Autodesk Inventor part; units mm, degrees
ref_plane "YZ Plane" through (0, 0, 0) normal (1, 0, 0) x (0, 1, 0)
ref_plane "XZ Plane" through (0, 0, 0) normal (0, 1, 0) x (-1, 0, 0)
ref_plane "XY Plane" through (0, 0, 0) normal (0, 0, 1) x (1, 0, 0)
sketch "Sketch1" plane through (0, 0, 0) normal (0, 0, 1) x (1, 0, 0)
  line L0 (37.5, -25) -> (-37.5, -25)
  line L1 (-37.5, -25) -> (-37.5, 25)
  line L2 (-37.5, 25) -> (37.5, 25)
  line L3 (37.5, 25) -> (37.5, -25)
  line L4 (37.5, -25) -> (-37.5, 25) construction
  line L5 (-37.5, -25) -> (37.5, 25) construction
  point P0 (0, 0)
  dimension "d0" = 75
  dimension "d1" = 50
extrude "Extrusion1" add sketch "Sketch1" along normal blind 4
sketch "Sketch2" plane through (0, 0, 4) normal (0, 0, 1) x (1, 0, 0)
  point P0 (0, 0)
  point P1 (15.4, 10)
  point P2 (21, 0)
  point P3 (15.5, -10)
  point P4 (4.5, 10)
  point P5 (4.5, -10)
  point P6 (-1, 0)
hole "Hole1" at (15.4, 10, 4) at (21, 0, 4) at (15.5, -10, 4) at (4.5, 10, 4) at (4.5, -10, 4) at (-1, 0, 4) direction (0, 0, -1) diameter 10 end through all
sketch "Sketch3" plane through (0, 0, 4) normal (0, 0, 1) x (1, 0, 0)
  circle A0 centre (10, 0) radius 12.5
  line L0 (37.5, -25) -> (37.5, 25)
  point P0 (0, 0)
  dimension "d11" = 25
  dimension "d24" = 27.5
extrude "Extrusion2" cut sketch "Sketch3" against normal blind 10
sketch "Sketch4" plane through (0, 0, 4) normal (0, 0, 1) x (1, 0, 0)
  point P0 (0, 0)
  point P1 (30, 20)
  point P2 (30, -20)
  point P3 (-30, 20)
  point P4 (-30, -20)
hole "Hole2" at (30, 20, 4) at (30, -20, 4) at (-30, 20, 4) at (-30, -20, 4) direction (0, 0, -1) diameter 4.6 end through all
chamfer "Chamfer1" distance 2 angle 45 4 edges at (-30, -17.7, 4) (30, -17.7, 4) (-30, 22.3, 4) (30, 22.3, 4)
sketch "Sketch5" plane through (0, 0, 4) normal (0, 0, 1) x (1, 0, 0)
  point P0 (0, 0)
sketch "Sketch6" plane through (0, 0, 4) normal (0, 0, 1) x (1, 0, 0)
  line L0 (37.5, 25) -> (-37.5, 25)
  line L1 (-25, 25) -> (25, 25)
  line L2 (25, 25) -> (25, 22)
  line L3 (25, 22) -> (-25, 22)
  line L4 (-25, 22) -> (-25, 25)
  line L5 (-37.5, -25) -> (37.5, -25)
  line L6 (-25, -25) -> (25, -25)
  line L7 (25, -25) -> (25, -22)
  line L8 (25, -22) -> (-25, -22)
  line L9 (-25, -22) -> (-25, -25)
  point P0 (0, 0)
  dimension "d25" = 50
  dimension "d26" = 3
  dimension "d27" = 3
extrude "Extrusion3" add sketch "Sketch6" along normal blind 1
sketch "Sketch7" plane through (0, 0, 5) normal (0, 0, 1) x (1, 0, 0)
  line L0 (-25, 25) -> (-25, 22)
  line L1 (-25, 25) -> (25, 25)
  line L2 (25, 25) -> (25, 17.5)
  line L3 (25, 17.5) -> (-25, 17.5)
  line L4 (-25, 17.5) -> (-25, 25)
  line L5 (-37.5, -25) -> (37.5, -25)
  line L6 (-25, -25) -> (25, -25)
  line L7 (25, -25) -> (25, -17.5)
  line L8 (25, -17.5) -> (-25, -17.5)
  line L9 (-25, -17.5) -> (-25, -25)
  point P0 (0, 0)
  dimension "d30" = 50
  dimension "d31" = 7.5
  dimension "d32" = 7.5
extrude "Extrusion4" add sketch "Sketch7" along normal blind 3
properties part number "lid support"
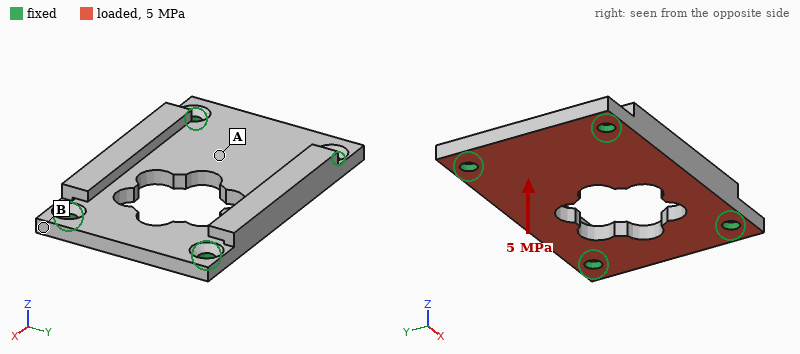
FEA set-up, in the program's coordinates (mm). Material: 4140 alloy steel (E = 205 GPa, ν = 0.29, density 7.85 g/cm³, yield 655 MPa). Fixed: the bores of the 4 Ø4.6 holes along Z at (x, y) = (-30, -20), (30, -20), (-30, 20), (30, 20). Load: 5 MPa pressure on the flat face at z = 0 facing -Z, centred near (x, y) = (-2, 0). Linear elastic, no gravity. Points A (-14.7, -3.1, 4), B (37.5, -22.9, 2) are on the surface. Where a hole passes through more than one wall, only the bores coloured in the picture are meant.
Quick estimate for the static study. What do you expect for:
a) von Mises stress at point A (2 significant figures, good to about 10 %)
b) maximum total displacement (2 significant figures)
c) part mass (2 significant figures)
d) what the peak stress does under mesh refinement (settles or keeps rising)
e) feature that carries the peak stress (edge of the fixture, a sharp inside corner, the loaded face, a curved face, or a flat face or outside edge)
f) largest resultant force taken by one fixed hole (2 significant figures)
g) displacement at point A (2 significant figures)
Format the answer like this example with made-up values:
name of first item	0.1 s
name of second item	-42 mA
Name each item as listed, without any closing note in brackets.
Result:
von Mises stress at point A	190 MPa
maximum total displacement	0.20 mm
part mass	110 g
what the peak stress does under mesh refinement	keeps rising
feature that carries the peak stress	edge of the fixture
largest resultant force taken by one fixed hole	5.1 kN
displacement at point A	0.14 mm
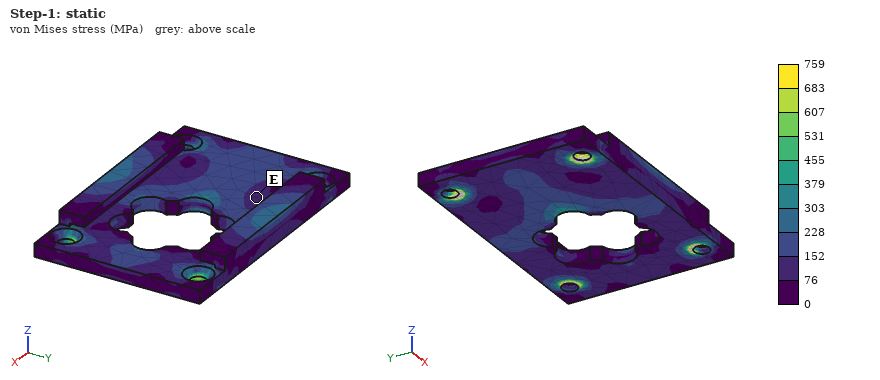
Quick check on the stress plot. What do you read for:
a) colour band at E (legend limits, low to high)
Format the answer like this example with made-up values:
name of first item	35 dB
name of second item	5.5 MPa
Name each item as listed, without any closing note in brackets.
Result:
colour band at E	76 to 152 MPa
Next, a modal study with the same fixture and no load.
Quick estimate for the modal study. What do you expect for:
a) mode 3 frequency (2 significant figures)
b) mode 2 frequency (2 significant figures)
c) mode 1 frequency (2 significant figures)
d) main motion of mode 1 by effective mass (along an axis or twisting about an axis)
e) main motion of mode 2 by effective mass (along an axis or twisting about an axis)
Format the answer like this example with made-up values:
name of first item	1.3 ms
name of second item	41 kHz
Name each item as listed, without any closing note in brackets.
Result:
mode 3 frequency	9600 Hz
mode 2 frequency	7900 Hz
mode 1 frequency	5700 Hz
main motion of mode 1 by effective mass	along Z
main motion of mode 2 by effective mass	twisting about X
